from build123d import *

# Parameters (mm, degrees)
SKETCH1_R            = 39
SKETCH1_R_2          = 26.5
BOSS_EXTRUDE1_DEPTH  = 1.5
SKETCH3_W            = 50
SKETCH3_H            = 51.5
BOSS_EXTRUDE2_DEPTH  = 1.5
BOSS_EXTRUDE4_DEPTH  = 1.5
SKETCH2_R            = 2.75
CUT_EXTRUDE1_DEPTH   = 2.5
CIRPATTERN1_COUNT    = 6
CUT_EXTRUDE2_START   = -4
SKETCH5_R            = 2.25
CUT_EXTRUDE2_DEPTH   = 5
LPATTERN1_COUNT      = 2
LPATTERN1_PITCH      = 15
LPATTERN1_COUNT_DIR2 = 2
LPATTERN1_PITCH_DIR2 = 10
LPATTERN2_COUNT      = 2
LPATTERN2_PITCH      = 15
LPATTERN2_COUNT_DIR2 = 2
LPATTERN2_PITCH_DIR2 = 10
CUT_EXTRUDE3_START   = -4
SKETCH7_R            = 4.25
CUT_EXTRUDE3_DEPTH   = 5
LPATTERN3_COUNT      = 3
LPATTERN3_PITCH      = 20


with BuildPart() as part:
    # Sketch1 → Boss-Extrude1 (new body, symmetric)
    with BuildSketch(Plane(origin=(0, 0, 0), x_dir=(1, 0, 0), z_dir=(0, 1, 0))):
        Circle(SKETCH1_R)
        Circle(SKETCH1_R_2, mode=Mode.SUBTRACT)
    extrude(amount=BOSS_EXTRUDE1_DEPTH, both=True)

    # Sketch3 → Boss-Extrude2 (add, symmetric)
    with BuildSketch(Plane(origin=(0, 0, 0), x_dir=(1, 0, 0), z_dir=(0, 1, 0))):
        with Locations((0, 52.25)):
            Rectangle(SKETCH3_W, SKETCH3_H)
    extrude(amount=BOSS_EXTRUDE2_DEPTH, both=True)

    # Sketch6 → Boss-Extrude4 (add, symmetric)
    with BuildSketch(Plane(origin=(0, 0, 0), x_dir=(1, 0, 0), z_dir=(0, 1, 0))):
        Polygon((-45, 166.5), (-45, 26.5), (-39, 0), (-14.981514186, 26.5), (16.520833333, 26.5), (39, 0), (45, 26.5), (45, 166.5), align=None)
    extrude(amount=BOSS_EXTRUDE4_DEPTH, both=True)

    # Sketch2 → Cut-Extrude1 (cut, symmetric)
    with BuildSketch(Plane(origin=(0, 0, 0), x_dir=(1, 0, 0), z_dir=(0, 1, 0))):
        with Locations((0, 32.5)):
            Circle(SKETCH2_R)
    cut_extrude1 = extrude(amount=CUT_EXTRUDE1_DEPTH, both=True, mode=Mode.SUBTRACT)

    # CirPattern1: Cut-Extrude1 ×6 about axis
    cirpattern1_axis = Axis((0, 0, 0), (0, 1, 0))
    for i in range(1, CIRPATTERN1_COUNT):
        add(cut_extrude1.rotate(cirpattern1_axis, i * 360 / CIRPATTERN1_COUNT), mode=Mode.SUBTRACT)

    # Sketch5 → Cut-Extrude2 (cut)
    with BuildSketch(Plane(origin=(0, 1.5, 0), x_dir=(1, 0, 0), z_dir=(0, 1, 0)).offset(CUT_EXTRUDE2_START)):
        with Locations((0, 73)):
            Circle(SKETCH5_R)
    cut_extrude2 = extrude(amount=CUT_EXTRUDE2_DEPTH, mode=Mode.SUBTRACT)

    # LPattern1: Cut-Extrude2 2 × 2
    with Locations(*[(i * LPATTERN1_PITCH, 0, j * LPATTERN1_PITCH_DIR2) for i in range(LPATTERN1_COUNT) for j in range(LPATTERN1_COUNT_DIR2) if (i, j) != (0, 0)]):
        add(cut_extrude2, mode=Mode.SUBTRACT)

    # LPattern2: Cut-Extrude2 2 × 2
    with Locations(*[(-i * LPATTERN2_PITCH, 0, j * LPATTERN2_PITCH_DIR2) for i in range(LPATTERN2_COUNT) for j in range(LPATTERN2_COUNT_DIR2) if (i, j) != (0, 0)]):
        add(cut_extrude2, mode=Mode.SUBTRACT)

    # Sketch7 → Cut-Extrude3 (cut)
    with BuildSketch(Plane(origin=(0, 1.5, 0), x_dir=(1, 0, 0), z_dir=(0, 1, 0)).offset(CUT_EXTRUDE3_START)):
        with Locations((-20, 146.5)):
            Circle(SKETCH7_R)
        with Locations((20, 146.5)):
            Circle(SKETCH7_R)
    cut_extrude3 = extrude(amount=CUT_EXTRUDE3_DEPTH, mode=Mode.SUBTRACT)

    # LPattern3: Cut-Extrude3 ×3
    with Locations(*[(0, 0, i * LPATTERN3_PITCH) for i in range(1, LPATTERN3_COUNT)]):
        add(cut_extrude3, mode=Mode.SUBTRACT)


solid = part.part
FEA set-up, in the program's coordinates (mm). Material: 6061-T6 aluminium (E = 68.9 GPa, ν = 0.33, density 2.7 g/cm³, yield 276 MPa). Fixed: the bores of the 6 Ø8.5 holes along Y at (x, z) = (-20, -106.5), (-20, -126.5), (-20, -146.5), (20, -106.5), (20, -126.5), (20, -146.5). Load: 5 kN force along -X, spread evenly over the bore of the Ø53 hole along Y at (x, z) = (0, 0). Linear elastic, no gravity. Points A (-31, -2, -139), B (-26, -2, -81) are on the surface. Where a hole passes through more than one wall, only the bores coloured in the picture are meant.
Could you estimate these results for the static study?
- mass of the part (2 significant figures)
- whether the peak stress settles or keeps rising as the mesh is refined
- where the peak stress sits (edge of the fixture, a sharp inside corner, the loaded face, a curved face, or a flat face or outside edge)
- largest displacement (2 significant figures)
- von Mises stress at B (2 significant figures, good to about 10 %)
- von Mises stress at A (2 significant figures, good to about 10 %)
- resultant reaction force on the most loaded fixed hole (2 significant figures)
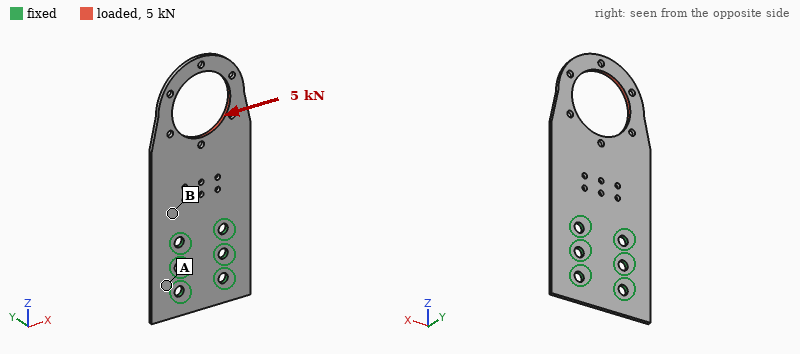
120 g
keeps rising
edge of the fixture
0.70 mm
69 MPa
35 MPa
7.5 kN
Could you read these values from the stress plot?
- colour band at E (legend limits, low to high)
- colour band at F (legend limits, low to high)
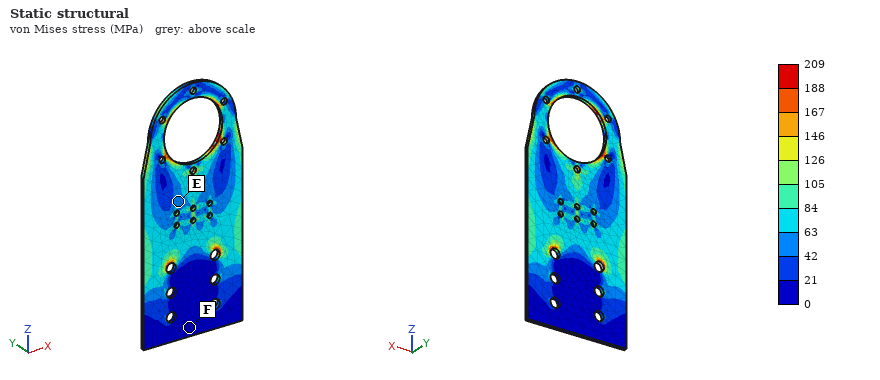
42 to 63 MPa
0 to 21 MPa
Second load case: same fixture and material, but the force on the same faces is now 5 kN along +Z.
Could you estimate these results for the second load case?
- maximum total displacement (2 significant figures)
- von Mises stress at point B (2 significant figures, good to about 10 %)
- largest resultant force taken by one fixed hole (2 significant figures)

0.10 mm
22 MPa
1.8 kN
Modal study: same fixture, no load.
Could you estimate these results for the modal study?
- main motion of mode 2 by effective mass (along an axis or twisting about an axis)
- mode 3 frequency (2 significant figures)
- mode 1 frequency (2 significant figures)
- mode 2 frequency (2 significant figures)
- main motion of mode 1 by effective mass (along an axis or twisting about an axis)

twisting about Z
700 Hz
180 Hz
520 Hz
along Y
